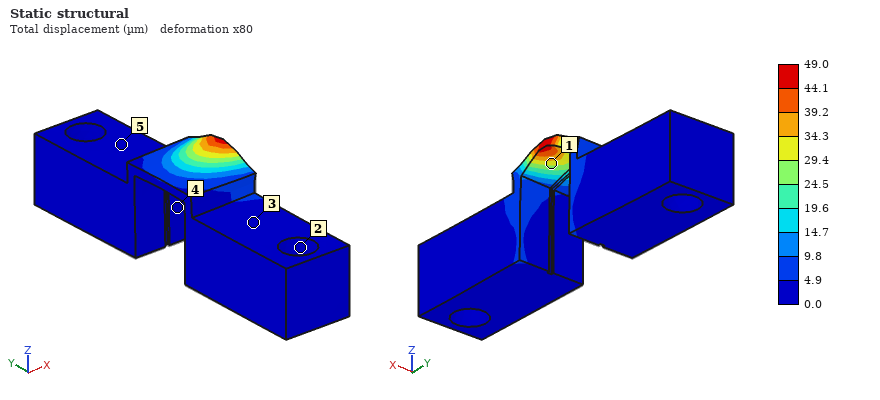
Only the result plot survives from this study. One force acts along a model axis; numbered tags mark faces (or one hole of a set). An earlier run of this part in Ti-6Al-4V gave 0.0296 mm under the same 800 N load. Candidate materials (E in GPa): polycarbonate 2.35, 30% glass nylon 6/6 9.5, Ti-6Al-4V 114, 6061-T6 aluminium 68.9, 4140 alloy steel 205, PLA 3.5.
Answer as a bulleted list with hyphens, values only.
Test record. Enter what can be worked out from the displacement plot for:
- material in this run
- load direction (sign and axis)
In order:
- 6061-T6 aluminium
- +Z
